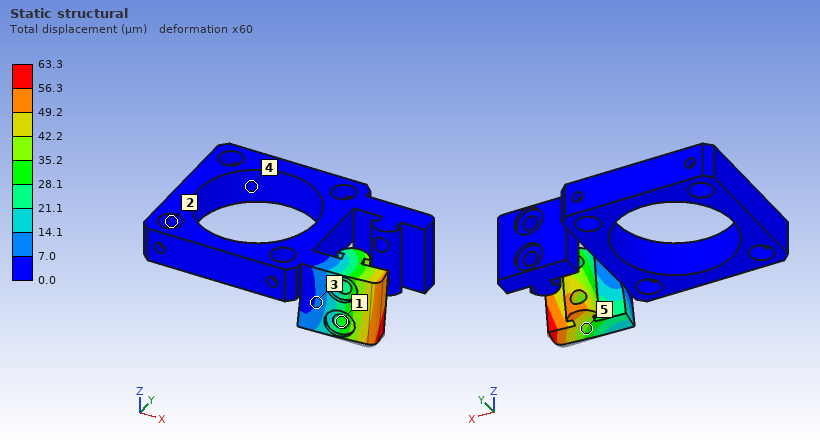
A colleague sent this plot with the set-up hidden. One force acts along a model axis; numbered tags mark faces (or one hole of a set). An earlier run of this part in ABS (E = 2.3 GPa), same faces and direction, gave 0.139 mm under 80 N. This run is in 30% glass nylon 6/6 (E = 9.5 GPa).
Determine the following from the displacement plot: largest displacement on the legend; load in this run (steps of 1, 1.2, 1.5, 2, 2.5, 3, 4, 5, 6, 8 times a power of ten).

63.3 µm
150 N
